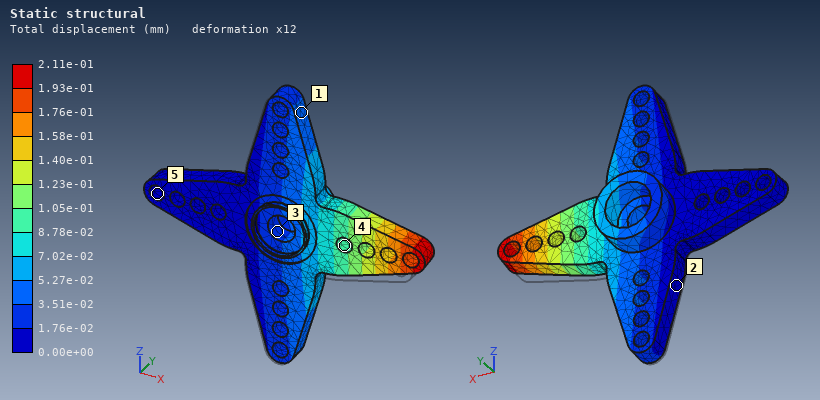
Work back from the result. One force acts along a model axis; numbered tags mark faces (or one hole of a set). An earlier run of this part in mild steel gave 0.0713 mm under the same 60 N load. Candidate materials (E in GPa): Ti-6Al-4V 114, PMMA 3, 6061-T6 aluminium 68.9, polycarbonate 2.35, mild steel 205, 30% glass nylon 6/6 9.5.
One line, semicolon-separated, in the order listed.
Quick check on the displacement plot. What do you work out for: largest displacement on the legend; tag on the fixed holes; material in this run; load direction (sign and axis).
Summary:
2.11e-01 mm; 5; 6061-T6 aluminium; +Y
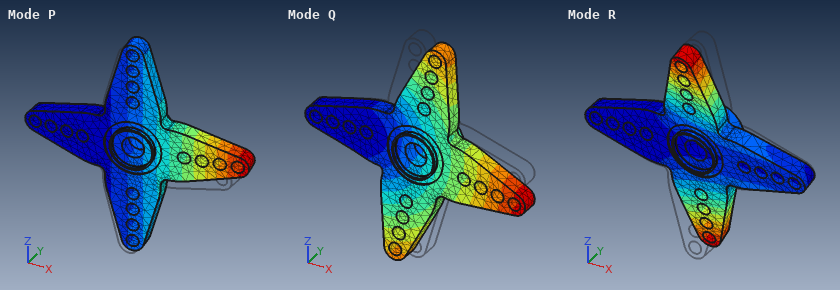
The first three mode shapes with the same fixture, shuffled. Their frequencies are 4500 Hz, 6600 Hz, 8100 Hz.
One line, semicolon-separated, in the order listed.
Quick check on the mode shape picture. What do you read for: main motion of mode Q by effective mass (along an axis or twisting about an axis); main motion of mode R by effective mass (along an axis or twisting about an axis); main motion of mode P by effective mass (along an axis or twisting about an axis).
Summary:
along Z; twisting about X; along Y
